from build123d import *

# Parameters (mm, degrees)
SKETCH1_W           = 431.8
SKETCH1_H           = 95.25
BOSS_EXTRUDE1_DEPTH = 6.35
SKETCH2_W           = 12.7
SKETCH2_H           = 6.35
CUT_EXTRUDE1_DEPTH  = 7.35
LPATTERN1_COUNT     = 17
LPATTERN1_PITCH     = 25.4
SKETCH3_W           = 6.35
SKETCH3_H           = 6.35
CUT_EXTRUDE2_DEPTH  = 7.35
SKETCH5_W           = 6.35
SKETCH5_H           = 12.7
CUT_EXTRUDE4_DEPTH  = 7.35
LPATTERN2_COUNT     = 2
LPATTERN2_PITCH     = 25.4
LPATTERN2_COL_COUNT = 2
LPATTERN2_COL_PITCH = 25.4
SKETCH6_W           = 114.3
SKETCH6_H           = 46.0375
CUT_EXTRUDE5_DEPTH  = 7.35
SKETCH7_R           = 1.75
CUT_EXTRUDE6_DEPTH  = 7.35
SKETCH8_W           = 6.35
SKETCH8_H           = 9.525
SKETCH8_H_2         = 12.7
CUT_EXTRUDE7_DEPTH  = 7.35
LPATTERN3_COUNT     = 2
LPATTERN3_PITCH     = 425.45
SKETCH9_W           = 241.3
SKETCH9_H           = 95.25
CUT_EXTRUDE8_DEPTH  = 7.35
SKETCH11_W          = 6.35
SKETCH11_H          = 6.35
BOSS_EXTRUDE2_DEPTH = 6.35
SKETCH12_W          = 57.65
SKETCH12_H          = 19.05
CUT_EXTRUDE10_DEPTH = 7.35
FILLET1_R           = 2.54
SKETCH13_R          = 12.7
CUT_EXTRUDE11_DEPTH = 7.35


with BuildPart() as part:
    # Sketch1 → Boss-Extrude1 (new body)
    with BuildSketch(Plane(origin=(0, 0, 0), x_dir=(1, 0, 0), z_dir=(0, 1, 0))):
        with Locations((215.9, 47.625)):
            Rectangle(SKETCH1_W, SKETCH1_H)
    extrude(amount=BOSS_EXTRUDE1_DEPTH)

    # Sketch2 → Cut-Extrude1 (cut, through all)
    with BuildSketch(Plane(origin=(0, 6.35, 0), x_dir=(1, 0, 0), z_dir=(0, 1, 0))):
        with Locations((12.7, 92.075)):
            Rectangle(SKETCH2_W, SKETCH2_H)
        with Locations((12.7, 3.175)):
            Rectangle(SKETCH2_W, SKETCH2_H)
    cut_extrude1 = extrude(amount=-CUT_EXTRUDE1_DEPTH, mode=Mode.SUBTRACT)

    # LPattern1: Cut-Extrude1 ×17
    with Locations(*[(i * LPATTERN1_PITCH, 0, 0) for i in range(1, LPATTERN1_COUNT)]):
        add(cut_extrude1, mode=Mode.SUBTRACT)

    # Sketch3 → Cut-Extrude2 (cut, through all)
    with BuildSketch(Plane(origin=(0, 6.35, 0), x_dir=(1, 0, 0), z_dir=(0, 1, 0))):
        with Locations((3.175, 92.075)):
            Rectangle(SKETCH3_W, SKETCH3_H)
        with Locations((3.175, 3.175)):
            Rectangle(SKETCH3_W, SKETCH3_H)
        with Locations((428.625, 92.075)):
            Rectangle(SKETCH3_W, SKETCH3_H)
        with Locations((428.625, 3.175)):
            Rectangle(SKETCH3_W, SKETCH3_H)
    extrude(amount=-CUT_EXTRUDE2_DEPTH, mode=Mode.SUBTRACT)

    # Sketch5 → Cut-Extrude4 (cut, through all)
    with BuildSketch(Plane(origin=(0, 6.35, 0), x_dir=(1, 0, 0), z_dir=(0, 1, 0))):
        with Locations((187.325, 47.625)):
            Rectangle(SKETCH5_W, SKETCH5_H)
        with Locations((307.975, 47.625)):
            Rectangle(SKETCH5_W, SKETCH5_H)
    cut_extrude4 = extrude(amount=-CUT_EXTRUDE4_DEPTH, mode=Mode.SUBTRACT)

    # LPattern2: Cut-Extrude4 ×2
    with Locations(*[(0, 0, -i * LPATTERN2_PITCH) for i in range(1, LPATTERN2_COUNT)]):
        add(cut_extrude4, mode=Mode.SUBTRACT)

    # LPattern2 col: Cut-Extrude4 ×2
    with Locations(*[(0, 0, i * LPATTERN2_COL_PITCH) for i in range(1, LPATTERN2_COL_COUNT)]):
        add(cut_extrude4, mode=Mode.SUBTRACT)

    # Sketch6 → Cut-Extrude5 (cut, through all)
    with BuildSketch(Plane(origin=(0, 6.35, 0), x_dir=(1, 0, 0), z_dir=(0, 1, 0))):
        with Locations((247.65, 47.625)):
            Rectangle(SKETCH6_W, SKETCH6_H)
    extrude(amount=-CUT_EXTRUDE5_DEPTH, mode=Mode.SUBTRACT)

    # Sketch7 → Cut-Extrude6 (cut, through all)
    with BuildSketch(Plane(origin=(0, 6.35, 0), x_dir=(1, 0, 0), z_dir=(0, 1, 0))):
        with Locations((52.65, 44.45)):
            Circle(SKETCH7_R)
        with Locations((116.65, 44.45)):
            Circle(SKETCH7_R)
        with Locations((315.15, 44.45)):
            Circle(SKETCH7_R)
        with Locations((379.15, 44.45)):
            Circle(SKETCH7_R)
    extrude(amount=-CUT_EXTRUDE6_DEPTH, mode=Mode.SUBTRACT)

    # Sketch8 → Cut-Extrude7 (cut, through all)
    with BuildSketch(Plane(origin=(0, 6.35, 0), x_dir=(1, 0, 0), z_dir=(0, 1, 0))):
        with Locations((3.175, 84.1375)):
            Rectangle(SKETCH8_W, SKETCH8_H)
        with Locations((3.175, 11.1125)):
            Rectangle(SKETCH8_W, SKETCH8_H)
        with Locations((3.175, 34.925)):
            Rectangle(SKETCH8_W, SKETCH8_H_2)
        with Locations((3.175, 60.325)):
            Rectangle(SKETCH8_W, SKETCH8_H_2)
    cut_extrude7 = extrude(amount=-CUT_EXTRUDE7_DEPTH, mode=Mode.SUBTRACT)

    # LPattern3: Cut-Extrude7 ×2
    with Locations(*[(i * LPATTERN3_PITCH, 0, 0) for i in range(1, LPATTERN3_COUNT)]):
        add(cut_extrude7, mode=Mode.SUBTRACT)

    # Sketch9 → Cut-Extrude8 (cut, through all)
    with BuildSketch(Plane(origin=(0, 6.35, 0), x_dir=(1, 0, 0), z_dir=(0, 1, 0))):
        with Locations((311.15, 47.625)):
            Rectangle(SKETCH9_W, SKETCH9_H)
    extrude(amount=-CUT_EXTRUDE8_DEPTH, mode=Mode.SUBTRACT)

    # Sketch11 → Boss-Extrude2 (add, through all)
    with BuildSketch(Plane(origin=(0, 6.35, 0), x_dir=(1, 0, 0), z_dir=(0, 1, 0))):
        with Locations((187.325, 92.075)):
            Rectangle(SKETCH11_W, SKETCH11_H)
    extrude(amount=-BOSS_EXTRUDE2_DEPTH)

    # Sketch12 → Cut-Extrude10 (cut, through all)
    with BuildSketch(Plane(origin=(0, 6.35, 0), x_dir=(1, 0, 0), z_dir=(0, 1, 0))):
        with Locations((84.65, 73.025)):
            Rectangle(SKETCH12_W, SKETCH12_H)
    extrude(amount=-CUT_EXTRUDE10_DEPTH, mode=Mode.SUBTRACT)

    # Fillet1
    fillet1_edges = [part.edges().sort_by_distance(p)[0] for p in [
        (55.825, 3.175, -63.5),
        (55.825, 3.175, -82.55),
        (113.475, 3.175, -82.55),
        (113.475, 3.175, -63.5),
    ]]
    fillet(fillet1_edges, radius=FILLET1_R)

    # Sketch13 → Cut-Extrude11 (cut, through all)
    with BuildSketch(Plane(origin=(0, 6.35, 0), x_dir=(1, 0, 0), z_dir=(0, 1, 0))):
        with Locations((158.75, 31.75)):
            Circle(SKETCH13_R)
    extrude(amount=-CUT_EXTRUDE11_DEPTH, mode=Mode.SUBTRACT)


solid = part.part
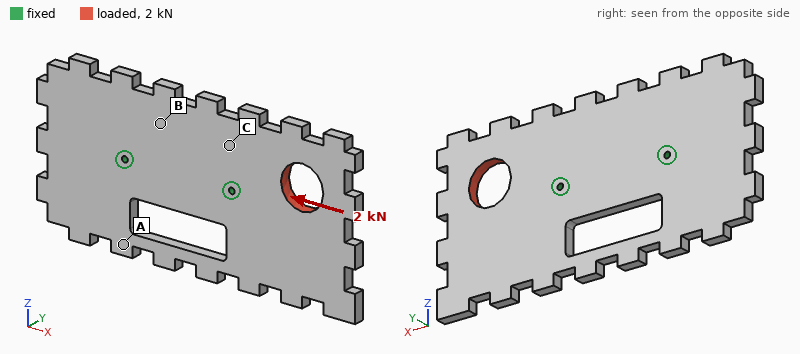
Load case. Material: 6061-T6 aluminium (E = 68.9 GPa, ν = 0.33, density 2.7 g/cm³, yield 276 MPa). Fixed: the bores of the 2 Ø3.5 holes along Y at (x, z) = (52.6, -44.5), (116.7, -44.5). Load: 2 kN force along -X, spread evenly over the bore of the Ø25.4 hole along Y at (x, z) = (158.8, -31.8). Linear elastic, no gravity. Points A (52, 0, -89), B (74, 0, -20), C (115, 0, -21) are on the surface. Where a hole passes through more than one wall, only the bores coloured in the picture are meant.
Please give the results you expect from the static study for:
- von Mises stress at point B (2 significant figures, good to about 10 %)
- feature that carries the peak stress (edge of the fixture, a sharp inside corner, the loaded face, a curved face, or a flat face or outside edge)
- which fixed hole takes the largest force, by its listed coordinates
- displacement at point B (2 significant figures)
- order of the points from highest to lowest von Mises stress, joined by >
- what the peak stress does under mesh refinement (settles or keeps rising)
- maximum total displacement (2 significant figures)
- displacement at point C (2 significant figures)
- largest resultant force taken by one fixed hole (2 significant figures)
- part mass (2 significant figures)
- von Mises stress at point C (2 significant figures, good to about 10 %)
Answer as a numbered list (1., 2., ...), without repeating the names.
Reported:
1. 3.1 MPa
2. edge of the fixture
3. (116.7, -44.5)
4. 2.5 µm
5. C > B > A
6. keeps rising
7. 15 µm
8. 4.4 µm
9. 1.5 kN
10. 250 g
11. 5.0 MPa
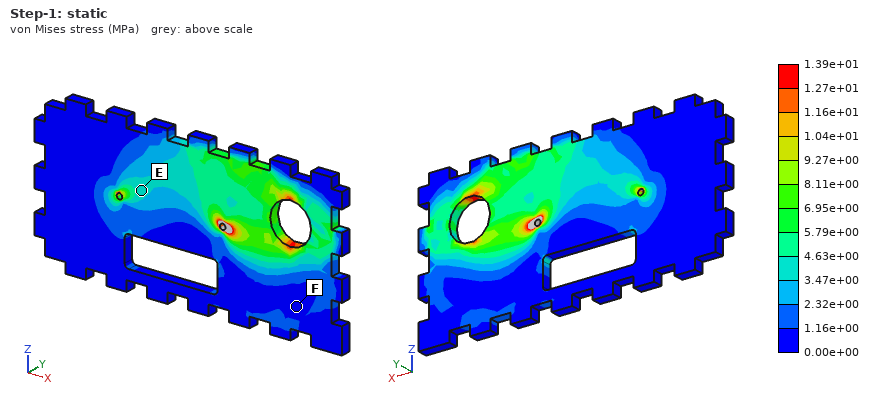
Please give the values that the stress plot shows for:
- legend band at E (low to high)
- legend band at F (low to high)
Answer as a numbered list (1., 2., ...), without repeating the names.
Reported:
1. 3.47e+00 to 4.63e+00 MPa
2. 0.00e+00 to 1.16e+00 MPa
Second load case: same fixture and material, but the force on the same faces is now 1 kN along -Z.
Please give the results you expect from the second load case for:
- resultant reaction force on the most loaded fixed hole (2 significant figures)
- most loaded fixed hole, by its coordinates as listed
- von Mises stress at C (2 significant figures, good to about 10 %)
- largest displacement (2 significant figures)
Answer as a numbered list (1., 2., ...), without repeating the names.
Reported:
1. 1.6 kN
2. (116.7, -44.5)
3. 4.4 MPa
4. 32 µm
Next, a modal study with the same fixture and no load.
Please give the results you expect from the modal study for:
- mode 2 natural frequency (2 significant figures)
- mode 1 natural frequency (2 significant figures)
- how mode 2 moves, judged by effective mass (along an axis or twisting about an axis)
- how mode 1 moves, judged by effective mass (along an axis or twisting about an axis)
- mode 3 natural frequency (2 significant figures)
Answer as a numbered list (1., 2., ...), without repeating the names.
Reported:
1. 1100 Hz
2. 760 Hz
3. twisting about X
4. along Y
5. 1300 Hz
